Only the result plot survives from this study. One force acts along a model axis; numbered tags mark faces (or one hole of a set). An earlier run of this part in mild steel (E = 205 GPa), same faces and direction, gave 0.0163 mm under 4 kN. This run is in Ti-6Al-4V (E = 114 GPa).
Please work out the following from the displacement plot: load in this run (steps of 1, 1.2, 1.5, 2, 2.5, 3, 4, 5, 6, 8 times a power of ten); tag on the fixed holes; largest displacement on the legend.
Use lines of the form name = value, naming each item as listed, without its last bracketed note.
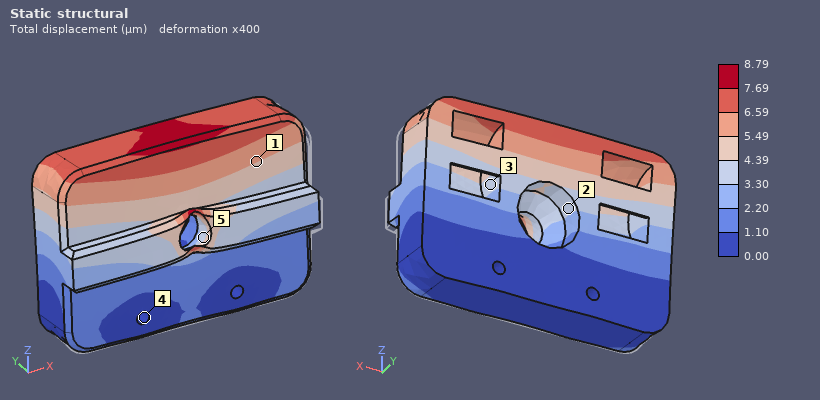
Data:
load in this run = 1.2 kN
tag on the fixed holes = 4
largest displacement on the legend = 8.79 µm
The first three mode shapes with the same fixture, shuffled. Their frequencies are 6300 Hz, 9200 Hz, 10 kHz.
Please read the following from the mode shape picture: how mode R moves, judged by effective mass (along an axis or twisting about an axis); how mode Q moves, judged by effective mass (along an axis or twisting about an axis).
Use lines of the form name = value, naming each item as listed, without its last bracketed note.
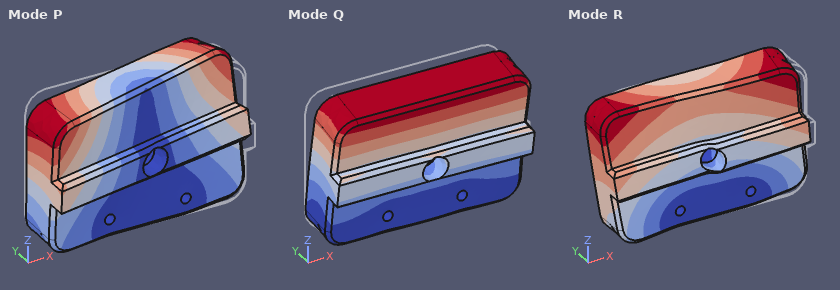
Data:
how mode R moves, judged by effective mass = along X
how mode Q moves, judged by effective mass = along Y
